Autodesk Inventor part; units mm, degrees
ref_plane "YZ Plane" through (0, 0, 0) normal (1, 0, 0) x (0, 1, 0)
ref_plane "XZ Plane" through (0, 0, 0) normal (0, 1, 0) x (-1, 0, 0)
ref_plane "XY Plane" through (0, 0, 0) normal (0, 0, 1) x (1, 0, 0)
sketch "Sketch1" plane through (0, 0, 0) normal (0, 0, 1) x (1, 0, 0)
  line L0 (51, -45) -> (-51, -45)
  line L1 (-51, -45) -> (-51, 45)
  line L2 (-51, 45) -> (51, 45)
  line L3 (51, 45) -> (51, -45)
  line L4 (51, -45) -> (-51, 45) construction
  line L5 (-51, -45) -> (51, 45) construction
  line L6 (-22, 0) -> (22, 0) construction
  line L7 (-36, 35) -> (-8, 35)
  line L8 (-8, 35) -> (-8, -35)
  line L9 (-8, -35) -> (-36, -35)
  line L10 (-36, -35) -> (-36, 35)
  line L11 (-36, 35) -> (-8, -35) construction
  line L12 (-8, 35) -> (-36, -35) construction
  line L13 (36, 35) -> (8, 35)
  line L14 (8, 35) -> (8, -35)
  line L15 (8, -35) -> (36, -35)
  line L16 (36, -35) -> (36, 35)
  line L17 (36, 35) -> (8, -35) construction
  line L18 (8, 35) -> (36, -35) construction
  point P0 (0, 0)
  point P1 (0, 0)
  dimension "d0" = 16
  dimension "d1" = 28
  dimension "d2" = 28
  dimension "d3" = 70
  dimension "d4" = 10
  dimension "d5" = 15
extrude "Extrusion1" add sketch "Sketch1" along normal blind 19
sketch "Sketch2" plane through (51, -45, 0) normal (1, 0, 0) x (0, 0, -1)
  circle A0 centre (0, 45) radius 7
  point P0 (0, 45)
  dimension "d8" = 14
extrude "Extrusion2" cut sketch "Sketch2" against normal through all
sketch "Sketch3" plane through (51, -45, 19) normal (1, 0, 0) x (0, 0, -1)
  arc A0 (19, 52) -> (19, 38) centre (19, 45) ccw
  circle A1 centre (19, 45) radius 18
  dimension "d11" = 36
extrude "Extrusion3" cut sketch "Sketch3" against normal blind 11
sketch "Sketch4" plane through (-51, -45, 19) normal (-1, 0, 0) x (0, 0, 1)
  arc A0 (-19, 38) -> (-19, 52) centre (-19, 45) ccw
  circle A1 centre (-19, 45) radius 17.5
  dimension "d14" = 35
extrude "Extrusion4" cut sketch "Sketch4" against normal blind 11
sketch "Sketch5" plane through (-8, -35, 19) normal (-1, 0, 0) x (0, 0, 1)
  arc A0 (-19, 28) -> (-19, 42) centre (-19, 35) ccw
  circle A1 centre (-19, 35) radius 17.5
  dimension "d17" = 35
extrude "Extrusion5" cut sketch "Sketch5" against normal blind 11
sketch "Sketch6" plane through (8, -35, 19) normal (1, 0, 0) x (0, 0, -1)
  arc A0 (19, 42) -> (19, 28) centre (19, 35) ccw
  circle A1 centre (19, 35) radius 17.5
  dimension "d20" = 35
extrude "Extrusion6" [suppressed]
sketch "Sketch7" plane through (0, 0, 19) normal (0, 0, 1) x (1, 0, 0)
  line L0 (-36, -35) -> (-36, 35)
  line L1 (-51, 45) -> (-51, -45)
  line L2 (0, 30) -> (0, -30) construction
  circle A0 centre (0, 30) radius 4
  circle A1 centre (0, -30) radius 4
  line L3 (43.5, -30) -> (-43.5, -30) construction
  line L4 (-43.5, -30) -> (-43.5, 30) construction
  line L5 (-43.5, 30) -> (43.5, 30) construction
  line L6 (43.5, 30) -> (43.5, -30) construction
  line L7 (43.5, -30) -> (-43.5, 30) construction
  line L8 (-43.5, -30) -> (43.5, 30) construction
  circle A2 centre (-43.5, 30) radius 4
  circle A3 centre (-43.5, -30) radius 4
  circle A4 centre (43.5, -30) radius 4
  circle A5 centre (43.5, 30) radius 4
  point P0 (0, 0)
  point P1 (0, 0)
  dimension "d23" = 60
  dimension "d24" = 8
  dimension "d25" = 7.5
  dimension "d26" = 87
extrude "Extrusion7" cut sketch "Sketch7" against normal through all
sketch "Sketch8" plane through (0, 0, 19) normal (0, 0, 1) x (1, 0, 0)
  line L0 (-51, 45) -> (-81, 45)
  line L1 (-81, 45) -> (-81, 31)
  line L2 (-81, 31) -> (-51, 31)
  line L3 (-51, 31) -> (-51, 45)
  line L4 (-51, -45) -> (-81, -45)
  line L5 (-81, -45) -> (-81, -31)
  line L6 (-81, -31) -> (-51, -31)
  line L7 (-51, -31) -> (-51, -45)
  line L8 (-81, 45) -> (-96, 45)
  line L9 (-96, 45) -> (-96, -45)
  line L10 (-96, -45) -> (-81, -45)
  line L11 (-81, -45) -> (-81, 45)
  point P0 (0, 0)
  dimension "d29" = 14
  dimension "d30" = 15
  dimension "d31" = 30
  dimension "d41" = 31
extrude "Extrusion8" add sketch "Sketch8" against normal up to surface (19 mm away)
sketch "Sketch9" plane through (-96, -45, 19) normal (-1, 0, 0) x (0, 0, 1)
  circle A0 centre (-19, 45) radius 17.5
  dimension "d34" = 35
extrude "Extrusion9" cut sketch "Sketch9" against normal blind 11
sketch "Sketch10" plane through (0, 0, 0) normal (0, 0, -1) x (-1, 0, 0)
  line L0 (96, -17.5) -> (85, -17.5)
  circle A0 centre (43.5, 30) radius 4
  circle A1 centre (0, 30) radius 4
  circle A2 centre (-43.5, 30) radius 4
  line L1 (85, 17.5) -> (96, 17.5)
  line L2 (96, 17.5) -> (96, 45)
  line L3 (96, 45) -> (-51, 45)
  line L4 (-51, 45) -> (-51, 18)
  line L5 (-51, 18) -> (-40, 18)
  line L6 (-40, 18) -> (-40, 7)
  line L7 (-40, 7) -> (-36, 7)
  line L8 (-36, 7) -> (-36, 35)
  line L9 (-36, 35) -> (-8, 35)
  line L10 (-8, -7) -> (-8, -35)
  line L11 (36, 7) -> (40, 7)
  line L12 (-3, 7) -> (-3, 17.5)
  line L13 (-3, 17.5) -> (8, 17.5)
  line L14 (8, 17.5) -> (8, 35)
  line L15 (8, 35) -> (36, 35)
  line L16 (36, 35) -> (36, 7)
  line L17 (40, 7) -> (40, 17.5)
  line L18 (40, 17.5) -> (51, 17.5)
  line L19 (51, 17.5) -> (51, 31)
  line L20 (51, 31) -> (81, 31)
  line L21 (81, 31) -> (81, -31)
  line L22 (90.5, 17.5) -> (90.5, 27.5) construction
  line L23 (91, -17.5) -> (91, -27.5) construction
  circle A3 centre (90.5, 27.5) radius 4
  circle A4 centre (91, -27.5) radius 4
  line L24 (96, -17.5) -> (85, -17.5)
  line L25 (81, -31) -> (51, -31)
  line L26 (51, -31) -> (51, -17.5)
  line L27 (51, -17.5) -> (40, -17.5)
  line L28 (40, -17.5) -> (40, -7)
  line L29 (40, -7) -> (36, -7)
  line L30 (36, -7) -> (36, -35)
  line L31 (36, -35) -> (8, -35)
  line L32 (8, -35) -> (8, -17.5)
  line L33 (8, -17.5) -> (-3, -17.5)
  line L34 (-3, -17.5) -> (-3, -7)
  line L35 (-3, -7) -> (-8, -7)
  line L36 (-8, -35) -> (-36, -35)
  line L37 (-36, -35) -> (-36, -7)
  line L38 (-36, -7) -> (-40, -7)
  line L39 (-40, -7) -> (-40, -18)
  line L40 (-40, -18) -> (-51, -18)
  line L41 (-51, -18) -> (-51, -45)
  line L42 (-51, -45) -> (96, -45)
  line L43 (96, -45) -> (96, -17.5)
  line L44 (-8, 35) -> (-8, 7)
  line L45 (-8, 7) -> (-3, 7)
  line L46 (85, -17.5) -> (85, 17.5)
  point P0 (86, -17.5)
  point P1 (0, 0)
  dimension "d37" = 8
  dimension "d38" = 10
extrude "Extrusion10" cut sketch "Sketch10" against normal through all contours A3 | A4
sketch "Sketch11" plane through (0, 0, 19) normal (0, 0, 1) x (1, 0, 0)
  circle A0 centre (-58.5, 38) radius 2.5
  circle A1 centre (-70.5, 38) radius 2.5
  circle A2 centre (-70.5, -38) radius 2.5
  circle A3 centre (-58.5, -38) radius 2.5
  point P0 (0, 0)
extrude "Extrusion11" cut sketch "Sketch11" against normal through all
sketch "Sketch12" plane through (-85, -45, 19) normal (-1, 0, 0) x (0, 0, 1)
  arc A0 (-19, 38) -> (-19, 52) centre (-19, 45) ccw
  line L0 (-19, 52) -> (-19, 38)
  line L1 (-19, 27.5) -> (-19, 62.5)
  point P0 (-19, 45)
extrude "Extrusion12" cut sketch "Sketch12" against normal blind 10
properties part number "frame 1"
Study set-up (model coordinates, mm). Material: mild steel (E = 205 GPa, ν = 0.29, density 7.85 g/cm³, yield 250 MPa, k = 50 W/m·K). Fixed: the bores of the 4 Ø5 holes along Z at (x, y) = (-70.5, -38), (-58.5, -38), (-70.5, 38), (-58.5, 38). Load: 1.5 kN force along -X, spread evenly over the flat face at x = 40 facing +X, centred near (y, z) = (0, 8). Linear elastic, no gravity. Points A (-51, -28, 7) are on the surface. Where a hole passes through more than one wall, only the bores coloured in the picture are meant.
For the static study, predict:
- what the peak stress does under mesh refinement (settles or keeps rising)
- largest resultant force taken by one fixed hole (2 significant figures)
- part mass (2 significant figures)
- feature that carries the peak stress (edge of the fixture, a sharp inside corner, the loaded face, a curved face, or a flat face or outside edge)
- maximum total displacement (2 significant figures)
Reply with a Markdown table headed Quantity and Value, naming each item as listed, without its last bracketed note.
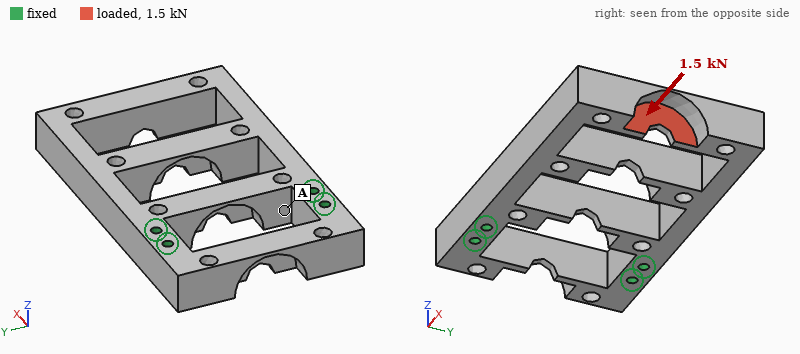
| Quantity | Value |
|---|---|
| what the peak stress does under mesh refinement | keeps rising |
| largest resultant force taken by one fixed hole | 670 N |
| part mass | 860 g |
| feature that carries the peak stress | a sharp inside corner |
| maximum total displacement | 35 µm |
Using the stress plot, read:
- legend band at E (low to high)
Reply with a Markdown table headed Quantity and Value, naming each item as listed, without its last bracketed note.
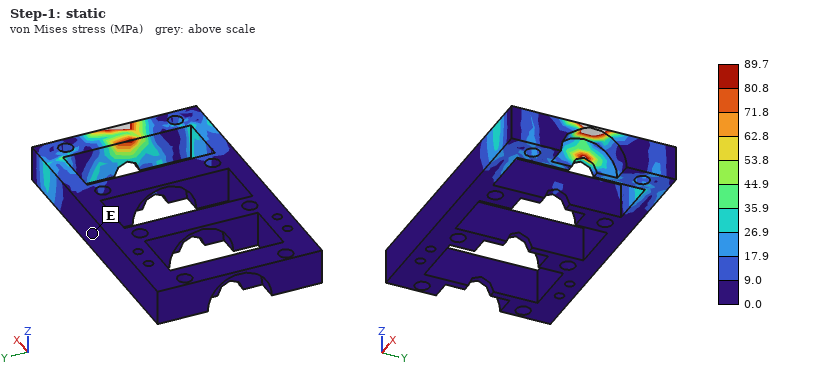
| Quantity | Value |
|---|---|
| legend band at E | 0.0 to 9.0 MPa |
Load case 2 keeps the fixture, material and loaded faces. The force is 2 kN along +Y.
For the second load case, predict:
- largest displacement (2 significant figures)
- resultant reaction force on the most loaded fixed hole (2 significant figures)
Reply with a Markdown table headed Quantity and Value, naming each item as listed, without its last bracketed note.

| Quantity | Value |
|---|---|
| largest displacement | 96 µm |
| resultant reaction force on the most loaded fixed hole | 2.5 kN |
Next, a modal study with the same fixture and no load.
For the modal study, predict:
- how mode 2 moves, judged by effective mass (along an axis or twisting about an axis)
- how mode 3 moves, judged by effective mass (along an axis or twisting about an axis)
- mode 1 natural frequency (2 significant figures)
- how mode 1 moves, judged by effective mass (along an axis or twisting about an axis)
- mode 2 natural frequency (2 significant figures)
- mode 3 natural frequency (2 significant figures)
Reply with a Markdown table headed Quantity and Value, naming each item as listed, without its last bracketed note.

| Quantity | Value |
|---|---|
| how mode 2 moves, judged by effective mass | along Y |
| how mode 3 moves, judged by effective mass | along Y |
| mode 1 natural frequency | 930 Hz |
| how mode 1 moves, judged by effective mass | along Z |
| mode 2 natural frequency | 1500 Hz |
| mode 3 natural frequency | 1700 Hz |
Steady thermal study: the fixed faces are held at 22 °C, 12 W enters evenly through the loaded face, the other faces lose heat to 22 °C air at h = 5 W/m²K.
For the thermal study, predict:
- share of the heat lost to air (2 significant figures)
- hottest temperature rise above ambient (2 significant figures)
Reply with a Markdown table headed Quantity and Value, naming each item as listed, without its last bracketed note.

| Quantity | Value |
|---|---|
| share of the heat lost to air | 29 % |
| hottest temperature rise above ambient | 68 K |
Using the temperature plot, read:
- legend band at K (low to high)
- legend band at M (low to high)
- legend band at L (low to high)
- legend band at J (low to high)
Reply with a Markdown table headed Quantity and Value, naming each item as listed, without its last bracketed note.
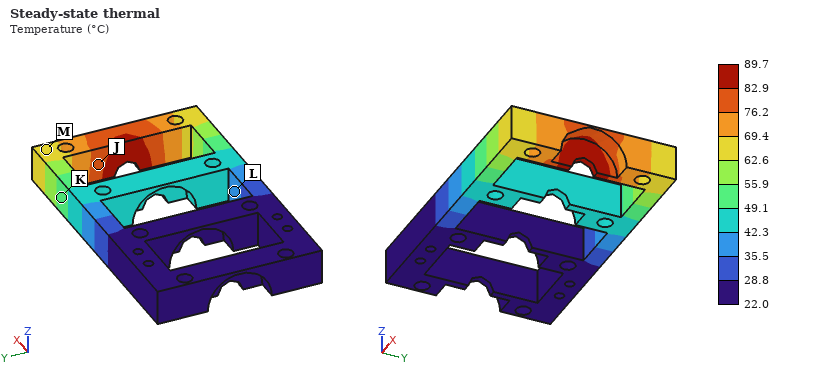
| Quantity | Value |
|---|---|
| legend band at K | 49.1 to 55.9 °C |
| legend band at M | 62.6 to 69.4 °C |
| legend band at L | 35.5 to 42.3 °C |
| legend band at J | 76.2 to 82.9 °C |
